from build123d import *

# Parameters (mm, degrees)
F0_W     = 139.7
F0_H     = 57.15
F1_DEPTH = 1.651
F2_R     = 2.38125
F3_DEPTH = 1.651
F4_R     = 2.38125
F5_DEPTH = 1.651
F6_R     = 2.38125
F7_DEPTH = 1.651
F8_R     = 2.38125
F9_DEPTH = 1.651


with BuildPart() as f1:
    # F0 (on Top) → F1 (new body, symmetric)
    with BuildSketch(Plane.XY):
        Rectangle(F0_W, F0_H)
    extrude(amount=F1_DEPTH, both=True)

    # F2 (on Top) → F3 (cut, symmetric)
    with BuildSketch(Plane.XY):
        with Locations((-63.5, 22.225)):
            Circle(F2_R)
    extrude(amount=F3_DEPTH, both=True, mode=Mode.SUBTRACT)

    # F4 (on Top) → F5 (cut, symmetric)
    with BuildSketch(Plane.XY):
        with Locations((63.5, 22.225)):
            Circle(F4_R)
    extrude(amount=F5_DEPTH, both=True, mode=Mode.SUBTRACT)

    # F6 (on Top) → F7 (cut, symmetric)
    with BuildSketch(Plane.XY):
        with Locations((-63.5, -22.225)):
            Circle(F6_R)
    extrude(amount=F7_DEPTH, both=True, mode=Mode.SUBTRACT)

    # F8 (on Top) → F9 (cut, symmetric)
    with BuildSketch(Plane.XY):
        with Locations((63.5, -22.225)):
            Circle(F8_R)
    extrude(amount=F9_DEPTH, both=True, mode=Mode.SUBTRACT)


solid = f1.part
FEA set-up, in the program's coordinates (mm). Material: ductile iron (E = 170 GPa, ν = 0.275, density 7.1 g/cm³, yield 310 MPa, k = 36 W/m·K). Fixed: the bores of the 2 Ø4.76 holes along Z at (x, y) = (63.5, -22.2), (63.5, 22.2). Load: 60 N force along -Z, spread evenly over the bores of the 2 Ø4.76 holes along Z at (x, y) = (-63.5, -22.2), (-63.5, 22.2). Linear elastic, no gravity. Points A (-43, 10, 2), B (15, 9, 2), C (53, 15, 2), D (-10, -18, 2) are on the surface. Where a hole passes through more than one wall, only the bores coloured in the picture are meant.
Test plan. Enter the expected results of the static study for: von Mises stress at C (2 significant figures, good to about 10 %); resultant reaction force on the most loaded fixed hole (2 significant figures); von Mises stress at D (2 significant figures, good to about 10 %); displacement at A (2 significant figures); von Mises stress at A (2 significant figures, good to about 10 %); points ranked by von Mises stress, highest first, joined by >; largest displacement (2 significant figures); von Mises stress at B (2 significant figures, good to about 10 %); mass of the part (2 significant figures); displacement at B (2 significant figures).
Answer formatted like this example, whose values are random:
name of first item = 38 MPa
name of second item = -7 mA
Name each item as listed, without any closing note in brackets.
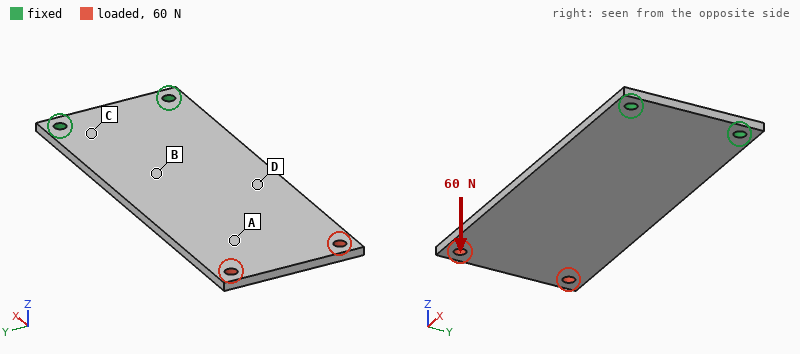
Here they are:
von Mises stress at C = 65 MPa
resultant reaction force on the most loaded fixed hole = 30 N
von Mises stress at D = 31 MPa
displacement at A = 1.1 mm
von Mises stress at A = 12 MPa
points ranked by von Mises stress, highest first, joined by > = C > B > D > A
largest displacement = 1.6 mm
von Mises stress at B = 45 MPa
mass of the part = 190 g
displacement at B = 0.30 mm
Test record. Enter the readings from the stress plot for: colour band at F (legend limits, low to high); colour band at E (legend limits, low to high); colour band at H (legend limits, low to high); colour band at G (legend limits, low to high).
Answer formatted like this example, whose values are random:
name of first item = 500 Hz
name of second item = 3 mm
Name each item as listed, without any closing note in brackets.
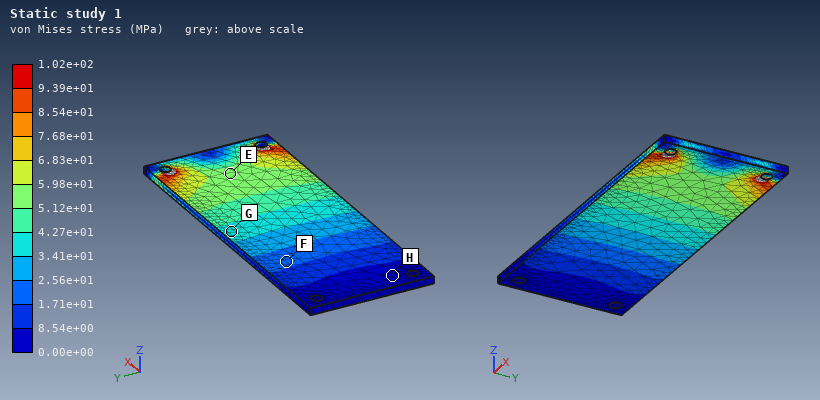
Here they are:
colour band at F = 1.71e+01 to 2.56e+01 MPa
colour band at E = 5.12e+01 to 5.98e+01 MPa
colour band at H = 0.00e+00 to 8.54e+00 MPa
colour band at G = 3.41e+01 to 4.27e+01 MPa
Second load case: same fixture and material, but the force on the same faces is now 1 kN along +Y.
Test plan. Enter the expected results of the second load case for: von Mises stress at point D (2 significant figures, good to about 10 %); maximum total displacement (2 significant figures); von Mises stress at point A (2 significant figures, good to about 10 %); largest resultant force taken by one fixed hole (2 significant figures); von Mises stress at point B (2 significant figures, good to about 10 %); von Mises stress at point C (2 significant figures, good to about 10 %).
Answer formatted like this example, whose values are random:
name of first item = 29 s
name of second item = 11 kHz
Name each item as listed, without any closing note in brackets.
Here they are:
von Mises stress at point D = 20 MPa
maximum total displacement = 0.10 mm
von Mises stress at point A = 13 MPa
largest resultant force taken by one fixed hole = 2.8 kN
von Mises stress at point B = 19 MPa
von Mises stress at point C = 34 MPa
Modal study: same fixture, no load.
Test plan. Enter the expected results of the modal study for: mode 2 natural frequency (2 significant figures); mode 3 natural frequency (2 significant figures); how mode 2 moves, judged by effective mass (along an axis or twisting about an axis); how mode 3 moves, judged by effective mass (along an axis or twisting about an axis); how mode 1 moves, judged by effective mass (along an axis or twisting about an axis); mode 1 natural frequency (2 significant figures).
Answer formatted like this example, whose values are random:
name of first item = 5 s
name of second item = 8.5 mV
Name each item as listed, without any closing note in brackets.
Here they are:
mode 2 natural frequency = 740 Hz
mode 3 natural frequency = 900 Hz
how mode 2 moves, judged by effective mass = twisting about X
how mode 3 moves, judged by effective mass = along Z
how mode 1 moves, judged by effective mass = along Z
mode 1 natural frequency = 140 Hz
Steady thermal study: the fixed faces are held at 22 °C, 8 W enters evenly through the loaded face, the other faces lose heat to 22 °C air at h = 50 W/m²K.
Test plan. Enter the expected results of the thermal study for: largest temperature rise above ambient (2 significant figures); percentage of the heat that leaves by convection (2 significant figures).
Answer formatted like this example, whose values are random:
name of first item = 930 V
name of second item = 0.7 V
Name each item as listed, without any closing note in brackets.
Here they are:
largest temperature rise above ambient = 44 K
percentage of the heat that leaves by convection = 97 %
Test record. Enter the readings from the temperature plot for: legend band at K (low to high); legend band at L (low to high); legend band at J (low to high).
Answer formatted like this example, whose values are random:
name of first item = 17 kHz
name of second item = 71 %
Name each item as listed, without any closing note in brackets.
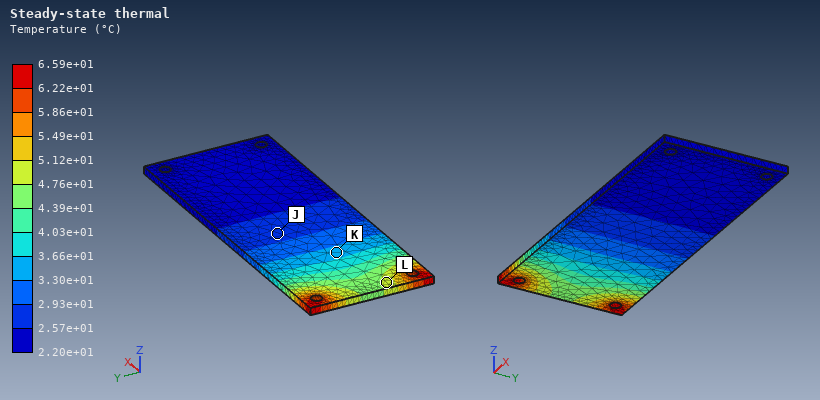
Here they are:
legend band at K = 3.30e+01 to 3.66e+01 °C
legend band at L = 4.76e+01 to 5.12e+01 °C
legend band at J = 2.57e+01 to 2.93e+01 °C
